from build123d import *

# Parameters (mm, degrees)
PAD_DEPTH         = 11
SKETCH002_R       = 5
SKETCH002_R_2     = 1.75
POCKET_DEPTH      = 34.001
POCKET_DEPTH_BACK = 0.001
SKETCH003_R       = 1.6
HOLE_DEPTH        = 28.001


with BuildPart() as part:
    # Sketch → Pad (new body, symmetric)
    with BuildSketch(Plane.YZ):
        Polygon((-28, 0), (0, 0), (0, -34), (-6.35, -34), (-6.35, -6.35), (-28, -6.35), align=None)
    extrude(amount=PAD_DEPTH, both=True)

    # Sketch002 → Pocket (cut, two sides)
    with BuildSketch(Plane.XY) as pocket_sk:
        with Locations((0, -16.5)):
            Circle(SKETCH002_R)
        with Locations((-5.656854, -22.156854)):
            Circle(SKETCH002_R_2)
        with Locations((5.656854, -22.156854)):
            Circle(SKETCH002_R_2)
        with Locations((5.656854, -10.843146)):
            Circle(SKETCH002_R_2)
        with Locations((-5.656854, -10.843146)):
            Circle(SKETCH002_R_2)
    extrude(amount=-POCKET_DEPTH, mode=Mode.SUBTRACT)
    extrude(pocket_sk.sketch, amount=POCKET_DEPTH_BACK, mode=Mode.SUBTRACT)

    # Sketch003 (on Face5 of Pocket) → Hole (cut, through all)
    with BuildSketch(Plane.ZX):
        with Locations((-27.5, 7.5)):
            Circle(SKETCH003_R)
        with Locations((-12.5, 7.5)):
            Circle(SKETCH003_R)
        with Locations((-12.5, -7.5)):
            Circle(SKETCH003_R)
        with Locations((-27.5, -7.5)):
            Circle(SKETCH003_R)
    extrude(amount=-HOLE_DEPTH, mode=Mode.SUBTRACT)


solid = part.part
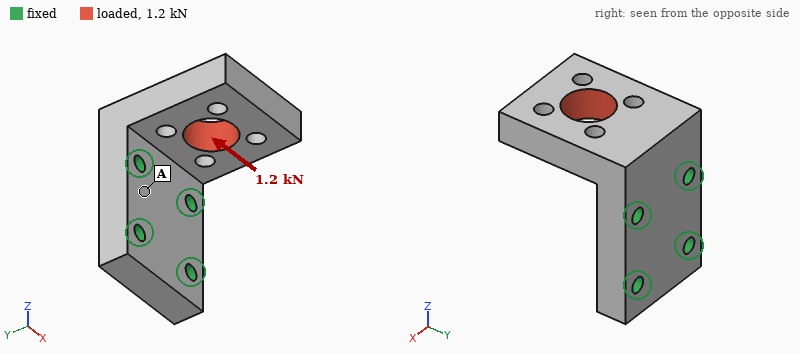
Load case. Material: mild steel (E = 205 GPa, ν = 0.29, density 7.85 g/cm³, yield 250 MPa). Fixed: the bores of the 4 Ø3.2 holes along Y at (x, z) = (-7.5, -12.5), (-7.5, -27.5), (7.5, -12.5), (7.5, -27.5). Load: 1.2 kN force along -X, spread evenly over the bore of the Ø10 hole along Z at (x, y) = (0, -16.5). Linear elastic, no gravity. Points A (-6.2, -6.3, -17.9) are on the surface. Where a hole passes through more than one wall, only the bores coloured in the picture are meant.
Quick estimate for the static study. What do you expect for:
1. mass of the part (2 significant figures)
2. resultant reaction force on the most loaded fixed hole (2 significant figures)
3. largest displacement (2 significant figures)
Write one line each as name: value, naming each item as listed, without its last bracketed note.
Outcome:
mass of the part: 54 g
resultant reaction force on the most loaded fixed hole: 1.2 kN
largest displacement: 19 µm
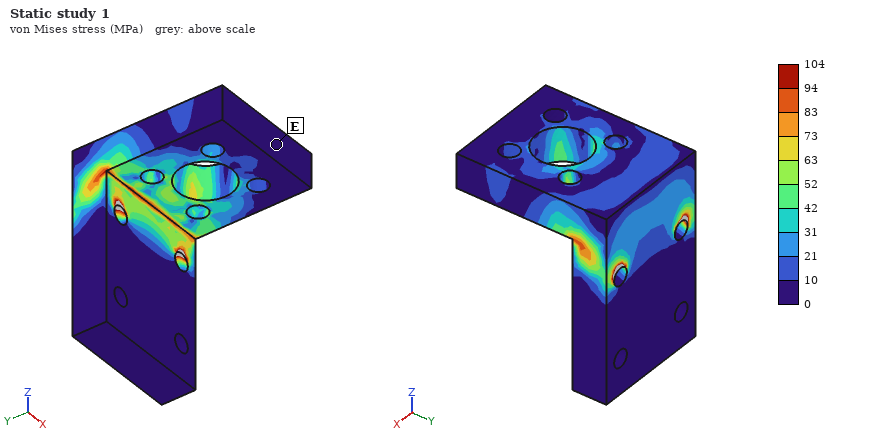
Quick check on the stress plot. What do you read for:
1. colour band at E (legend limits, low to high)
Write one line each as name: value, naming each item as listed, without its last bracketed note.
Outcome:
colour band at E: 0 to 10 MPa
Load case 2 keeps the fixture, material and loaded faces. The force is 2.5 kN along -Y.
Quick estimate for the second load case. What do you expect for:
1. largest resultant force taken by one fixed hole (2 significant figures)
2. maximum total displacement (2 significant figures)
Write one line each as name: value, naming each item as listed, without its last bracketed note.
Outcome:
largest resultant force taken by one fixed hole: 1.4 kN
maximum total displacement: 34 µm
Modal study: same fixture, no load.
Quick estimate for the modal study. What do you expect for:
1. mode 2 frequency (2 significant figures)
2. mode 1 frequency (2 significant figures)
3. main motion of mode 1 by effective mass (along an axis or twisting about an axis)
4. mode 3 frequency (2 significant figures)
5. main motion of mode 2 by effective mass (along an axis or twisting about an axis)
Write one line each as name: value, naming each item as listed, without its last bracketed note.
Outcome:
mode 2 frequency: 10 kHz
mode 1 frequency: 5500 Hz
main motion of mode 1 by effective mass: along Z
mode 3 frequency: 15 kHz
main motion of mode 2 by effective mass: along X
